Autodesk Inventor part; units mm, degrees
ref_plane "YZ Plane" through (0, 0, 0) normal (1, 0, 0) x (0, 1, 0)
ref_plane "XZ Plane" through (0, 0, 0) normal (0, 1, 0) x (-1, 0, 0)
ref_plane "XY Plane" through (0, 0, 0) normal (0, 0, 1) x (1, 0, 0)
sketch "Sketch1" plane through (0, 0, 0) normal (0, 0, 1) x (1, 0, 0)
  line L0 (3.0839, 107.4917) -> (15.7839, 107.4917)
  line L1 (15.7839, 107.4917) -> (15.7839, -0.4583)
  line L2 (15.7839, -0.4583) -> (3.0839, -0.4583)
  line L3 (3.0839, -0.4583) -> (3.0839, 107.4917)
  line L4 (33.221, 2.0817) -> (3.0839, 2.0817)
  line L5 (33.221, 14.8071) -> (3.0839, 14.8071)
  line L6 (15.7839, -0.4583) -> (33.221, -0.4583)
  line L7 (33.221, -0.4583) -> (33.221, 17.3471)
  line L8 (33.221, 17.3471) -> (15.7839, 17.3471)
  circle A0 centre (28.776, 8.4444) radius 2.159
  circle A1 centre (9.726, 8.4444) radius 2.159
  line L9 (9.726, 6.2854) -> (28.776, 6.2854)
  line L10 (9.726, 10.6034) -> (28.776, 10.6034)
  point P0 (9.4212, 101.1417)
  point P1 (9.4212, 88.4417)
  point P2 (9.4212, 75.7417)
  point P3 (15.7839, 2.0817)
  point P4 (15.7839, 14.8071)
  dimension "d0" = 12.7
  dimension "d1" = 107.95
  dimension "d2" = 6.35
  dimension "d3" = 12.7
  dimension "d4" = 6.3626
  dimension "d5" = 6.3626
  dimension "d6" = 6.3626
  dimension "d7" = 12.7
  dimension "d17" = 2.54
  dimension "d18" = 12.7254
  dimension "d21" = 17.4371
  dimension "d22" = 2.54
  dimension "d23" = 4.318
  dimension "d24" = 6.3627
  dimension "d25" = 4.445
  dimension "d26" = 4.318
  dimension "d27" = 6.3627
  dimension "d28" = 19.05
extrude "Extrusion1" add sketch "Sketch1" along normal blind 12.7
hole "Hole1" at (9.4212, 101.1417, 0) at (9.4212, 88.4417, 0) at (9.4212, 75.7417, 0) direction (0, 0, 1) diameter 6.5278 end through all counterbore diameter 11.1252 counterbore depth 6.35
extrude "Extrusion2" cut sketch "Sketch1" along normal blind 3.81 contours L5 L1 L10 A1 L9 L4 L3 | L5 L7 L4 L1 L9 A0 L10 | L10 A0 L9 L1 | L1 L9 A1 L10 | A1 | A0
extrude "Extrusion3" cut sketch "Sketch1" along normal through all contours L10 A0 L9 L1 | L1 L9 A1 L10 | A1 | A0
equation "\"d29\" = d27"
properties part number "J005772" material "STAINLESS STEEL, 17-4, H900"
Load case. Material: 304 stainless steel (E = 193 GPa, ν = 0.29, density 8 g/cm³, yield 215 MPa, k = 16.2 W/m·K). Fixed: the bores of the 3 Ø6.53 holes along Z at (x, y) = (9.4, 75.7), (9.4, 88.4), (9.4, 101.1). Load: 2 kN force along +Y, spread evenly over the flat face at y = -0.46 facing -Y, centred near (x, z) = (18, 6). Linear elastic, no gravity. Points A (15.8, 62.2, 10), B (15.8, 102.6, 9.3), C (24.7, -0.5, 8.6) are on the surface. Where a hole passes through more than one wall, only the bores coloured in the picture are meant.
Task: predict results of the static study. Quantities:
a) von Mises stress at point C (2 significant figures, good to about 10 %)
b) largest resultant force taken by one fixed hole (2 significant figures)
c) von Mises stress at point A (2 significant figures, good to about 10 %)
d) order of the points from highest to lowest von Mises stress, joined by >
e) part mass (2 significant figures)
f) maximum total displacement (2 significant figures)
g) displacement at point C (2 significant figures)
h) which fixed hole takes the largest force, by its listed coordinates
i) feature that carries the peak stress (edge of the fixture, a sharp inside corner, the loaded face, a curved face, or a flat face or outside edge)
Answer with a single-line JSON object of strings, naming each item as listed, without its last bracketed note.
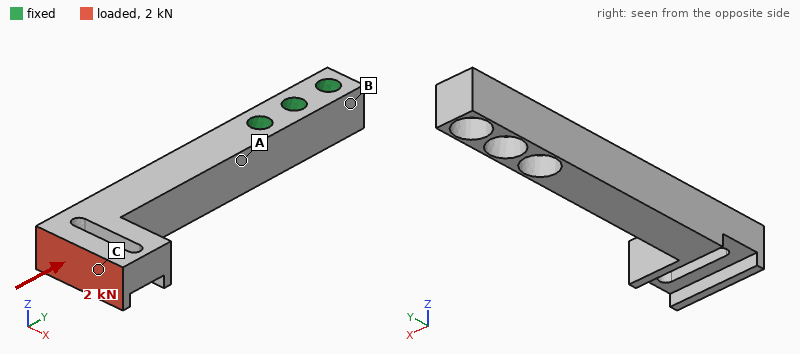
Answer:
{"von Mises stress at point C": "52 MPa", "largest resultant force taken by one fixed hole": "1.7 kN", "von Mises stress at point A": "70 MPa", "order of the points from highest to lowest von Mises stress, joined by >": "A > C > B", "part mass": "130 g", "maximum total displacement": "0.19 mm", "displacement at point C": "0.17 mm", "which fixed hole takes the largest force, by its listed coordinates": "(9.4, 75.7)", "feature that carries the peak stress": "a curved face"}
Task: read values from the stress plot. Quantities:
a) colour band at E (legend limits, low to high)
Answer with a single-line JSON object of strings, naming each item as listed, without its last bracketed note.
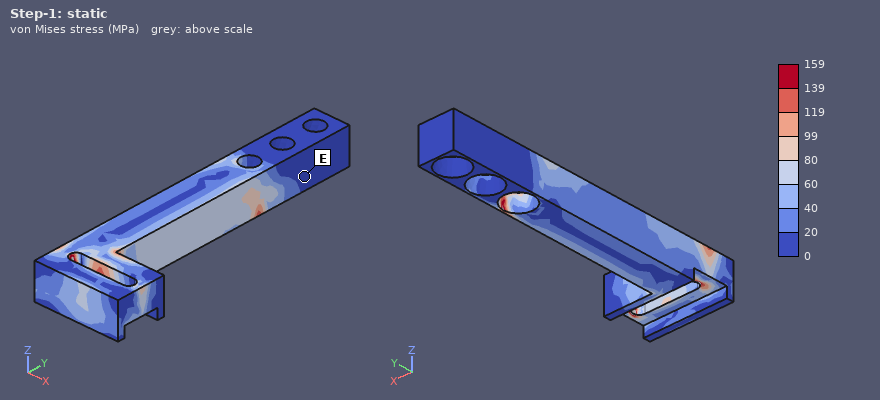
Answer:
{"colour band at E": "0 to 20 MPa"}
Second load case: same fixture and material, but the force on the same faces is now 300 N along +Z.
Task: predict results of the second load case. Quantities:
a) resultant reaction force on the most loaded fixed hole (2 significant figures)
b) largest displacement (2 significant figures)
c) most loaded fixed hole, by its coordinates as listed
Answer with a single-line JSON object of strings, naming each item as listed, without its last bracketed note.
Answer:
{"resultant reaction force on the most loaded fixed hole": "1.0 kN", "largest displacement": "0.19 mm", "most loaded fixed hole, by its coordinates as listed": "(9.4, 75.7)"}
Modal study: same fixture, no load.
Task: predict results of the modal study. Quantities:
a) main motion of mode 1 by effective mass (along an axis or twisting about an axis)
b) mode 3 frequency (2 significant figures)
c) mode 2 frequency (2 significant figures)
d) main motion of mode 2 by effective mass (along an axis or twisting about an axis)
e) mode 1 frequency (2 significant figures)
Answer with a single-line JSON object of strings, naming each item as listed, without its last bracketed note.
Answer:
{"main motion of mode 1 by effective mass": "along Z", "mode 3 frequency": "4400 Hz", "mode 2 frequency": "1300 Hz", "main motion of mode 2 by effective mass": "along X", "mode 1 frequency": "1100 Hz"}
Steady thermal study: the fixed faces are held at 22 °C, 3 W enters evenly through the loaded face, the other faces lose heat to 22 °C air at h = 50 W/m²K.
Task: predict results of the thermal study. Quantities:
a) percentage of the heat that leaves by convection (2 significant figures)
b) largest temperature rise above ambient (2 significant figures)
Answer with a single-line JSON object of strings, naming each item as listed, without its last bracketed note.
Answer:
{"percentage of the heat that leaves by convection": "91 %", "largest temperature rise above ambient": "33 K"}
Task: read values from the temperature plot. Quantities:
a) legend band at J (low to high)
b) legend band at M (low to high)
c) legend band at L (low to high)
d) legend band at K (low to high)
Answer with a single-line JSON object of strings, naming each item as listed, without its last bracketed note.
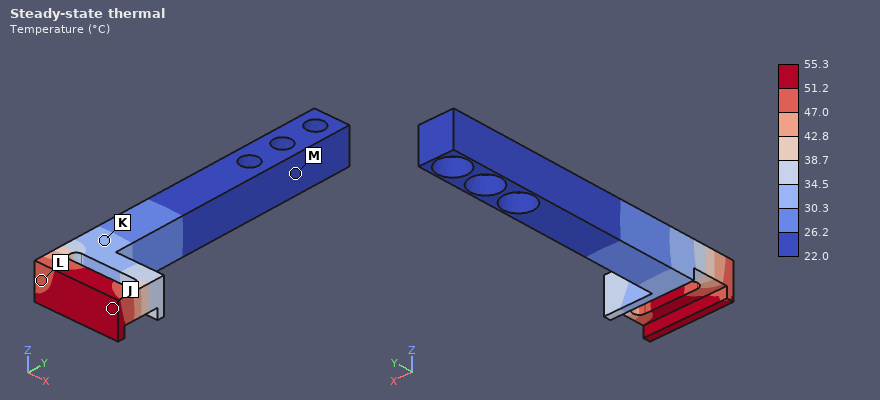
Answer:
{"legend band at J": "51.2 to 55.3 °C", "legend band at M": "22.0 to 26.2 °C", "legend band at L": "47.0 to 51.2 °C", "legend band at K": "30.3 to 34.5 °C"}
